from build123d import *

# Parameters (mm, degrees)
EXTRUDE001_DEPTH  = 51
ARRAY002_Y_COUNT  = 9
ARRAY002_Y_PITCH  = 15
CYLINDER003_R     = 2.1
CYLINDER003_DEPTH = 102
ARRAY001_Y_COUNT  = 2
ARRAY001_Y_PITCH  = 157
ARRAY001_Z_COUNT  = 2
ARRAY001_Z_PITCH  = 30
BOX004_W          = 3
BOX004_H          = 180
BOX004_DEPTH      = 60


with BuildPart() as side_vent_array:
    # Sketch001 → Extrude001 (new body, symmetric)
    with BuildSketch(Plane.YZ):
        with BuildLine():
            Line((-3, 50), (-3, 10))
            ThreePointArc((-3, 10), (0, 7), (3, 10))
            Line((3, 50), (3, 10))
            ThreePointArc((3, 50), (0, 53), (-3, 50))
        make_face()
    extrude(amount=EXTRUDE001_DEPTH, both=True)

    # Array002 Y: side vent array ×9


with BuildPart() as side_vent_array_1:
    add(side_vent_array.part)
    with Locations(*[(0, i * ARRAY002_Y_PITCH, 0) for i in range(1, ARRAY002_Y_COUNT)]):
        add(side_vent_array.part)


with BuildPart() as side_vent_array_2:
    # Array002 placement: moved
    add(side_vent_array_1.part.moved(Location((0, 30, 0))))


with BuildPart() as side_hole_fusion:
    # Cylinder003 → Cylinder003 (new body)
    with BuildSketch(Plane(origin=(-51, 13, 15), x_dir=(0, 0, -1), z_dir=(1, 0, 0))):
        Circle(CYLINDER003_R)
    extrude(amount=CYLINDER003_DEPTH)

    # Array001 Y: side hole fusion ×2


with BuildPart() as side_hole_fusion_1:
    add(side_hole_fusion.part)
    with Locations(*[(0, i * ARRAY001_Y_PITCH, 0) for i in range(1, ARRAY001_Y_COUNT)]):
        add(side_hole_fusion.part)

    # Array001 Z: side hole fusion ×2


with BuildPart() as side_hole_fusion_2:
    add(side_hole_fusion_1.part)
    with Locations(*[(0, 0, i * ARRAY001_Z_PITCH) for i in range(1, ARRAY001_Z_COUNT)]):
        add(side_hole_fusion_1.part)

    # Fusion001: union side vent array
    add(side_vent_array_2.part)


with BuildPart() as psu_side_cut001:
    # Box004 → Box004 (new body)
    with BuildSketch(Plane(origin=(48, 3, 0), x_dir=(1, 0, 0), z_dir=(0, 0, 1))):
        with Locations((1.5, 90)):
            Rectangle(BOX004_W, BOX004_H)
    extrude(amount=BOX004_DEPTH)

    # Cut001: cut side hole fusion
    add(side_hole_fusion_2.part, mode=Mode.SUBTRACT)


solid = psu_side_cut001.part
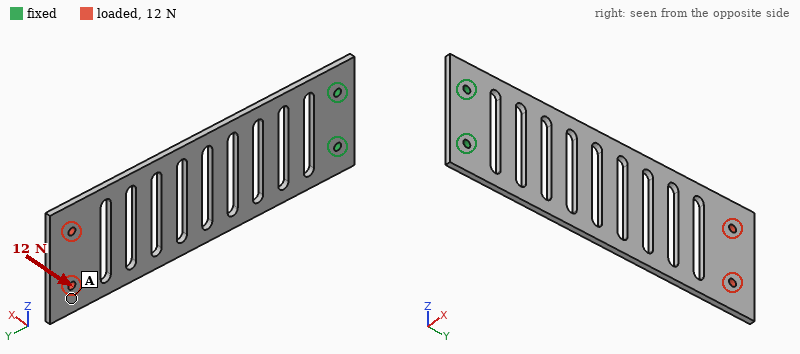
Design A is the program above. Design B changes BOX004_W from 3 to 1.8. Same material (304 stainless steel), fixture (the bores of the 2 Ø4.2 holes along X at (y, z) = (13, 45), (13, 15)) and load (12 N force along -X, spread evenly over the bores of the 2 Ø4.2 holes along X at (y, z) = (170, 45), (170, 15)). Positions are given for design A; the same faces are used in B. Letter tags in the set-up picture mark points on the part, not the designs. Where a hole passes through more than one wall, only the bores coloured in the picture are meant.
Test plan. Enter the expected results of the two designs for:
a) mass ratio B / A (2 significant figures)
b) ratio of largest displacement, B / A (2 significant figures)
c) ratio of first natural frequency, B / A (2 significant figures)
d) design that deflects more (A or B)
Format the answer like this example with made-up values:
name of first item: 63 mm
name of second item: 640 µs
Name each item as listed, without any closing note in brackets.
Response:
mass ratio B / A: 0.60
ratio of largest displacement, B / A: 4.5
ratio of first natural frequency, B / A: 0.61
design that deflects more: B
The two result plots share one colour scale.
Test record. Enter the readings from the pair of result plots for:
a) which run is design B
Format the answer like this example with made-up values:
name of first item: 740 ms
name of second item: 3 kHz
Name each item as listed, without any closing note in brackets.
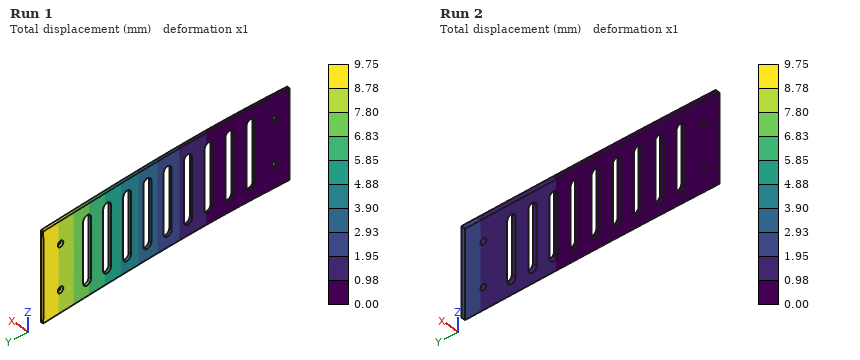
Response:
which run is design B: Run 1
